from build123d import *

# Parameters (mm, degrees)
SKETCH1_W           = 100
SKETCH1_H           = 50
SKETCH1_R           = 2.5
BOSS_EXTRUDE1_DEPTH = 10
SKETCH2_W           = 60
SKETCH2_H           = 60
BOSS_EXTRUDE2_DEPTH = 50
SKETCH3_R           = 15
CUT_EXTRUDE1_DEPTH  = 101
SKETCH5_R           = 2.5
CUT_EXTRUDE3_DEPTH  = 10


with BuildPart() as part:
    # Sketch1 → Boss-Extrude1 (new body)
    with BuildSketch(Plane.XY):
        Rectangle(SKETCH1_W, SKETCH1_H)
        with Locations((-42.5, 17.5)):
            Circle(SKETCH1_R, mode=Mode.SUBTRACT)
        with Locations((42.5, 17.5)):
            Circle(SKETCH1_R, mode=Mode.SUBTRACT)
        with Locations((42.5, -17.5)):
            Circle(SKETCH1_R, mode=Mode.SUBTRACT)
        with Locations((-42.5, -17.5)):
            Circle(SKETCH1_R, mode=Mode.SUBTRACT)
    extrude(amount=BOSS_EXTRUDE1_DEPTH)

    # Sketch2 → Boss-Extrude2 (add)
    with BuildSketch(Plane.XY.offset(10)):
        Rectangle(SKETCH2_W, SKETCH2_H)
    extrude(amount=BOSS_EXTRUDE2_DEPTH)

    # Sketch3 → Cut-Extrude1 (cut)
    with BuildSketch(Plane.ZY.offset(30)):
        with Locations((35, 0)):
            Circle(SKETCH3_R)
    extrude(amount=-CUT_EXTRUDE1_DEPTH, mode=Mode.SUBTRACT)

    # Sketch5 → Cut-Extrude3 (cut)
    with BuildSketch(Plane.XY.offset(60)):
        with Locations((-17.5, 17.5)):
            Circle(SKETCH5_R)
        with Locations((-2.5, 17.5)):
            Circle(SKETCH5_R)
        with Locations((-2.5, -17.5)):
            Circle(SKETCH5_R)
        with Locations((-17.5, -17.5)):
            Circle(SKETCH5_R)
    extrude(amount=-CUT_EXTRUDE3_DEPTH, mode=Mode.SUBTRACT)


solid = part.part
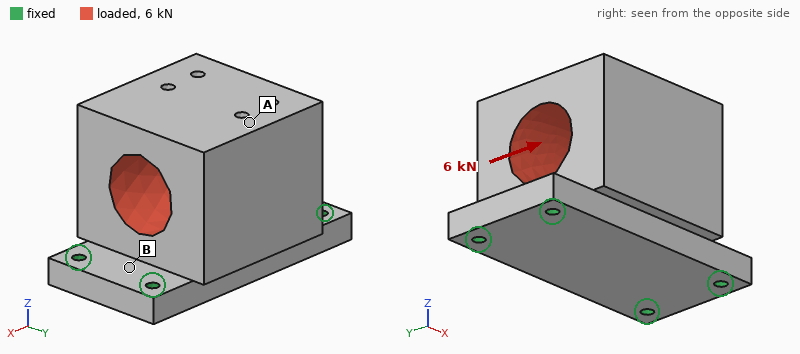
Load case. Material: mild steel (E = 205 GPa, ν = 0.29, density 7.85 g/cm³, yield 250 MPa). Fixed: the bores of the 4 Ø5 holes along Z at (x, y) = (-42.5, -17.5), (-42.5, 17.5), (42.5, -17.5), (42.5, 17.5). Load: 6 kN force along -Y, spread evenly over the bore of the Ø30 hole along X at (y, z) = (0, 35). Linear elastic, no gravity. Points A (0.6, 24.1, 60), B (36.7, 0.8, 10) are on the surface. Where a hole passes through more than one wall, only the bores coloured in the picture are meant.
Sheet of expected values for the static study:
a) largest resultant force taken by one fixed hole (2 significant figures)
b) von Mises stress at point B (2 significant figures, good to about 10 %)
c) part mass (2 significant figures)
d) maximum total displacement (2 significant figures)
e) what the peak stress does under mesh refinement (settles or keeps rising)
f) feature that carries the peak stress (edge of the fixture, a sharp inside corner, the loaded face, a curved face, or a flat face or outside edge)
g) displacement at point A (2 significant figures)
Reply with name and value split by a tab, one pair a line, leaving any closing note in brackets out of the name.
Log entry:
largest resultant force taken by one fixed hole	3.3 kN
von Mises stress at point B	30 MPa
part mass	1.5 kg
maximum total displacement	27 µm
what the peak stress does under mesh refinement	keeps rising
feature that carries the peak stress	edge of the fixture
displacement at point A	27 µm
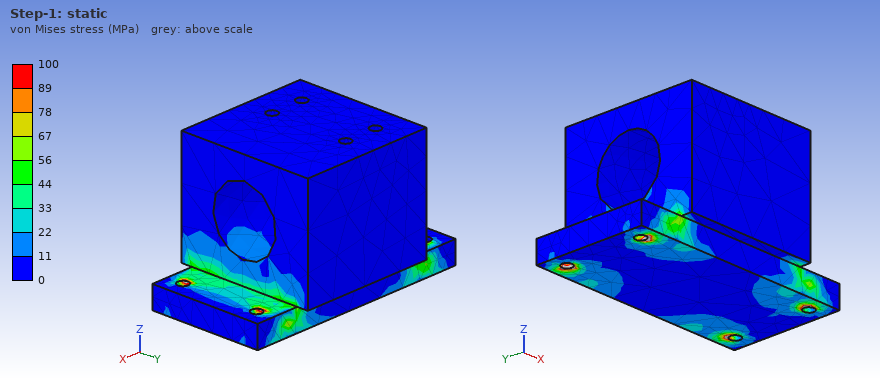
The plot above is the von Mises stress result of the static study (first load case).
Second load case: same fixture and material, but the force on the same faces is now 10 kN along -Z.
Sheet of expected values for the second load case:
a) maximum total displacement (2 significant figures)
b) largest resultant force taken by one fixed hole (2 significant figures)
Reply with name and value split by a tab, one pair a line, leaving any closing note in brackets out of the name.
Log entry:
maximum total displacement	8.4 µm
largest resultant force taken by one fixed hole	2.8 kN
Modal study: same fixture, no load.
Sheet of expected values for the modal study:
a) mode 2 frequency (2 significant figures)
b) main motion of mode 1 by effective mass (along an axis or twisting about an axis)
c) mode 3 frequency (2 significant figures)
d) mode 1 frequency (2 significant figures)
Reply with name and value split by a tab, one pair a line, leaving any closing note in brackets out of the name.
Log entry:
mode 2 frequency	5000 Hz
main motion of mode 1 by effective mass	along Y
mode 3 frequency	5200 Hz
mode 1 frequency	2500 Hz
